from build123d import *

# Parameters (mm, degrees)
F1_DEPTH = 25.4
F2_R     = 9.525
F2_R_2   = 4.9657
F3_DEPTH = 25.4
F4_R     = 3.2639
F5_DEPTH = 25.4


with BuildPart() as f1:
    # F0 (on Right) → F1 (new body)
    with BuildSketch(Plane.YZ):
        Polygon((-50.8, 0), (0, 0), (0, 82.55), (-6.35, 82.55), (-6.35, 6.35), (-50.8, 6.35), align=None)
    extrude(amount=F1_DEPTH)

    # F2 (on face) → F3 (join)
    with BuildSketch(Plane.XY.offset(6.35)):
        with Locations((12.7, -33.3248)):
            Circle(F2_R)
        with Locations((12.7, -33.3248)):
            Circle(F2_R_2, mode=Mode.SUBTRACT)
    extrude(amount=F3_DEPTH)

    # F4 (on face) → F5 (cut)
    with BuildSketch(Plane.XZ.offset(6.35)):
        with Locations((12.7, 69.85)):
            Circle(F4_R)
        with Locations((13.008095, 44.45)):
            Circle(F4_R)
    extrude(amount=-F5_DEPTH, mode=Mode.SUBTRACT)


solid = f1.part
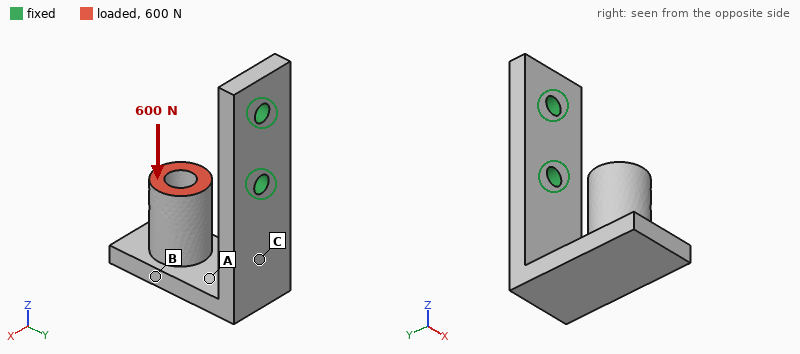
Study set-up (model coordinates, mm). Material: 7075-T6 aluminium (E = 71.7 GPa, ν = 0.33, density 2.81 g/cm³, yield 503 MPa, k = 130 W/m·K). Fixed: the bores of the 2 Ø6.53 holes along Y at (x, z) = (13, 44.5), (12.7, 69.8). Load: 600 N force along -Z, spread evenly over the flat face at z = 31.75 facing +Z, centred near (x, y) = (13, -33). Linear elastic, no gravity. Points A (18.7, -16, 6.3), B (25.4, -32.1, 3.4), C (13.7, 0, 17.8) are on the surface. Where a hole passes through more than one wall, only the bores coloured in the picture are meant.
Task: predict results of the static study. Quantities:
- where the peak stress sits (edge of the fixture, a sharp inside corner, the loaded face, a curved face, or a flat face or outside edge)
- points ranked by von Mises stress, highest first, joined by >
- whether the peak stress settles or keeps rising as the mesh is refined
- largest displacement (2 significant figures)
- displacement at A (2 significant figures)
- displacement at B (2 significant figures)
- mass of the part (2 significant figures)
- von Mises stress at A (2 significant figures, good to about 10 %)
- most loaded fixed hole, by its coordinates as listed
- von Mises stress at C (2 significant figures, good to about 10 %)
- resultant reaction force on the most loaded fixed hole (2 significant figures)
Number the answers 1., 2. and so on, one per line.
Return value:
1. edge of the fixture
2. C > A > B
3. keeps rising
4. 1.2 mm
5. 0.40 mm
6. 0.73 mm
7. 71 g
8. 59 MPa
9. (13, 44.5)
10. 94 MPa
11. 530 N
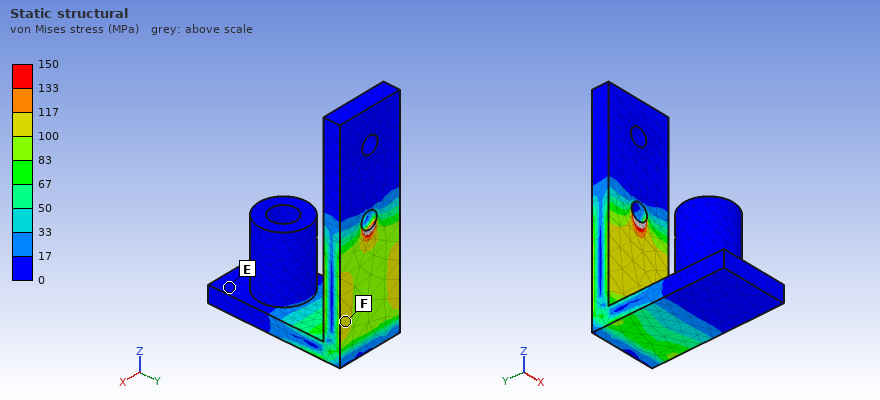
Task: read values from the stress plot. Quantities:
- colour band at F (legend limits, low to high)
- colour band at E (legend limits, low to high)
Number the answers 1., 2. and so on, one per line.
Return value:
1. 100 to 117 MPa
2. 0 to 17 MPa
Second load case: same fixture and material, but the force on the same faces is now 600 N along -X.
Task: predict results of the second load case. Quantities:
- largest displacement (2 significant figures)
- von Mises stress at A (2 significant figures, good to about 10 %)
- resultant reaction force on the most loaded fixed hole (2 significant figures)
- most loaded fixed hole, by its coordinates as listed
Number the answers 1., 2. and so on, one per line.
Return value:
1. 0.81 mm
2. 96 MPa
3. 760 N
4. (13, 44.5)
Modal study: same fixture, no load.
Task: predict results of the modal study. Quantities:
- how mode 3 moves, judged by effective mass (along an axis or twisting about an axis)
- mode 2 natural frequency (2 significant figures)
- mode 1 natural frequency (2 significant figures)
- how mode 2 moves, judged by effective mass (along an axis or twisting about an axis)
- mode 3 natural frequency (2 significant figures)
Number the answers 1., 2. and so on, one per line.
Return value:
1. along Y
2. 980 Hz
3. 720 Hz
4. along X
5. 1700 Hz
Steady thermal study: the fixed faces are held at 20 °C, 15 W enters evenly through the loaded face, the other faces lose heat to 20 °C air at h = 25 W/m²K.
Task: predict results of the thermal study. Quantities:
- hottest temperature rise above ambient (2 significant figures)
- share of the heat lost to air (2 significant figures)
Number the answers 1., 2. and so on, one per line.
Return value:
1. 46 K
2. 34 %
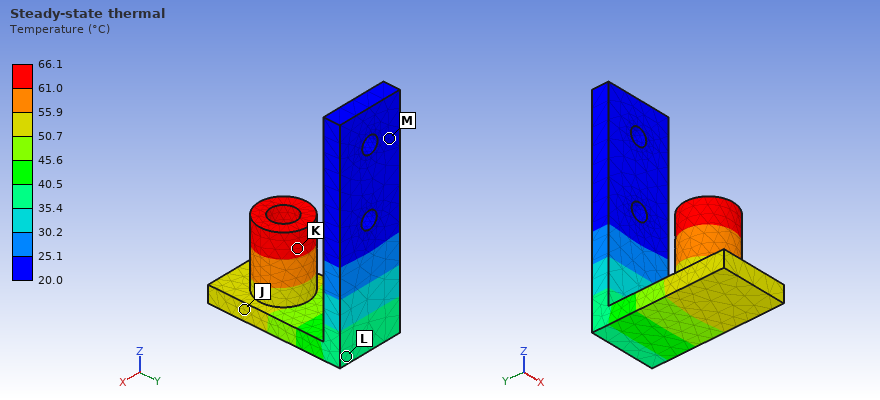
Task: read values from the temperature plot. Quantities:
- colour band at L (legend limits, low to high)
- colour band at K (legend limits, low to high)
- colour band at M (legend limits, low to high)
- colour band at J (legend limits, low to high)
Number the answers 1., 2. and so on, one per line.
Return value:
1. 35.4 to 40.5 °C
2. 61.0 to 66.1 °C
3. 20.0 to 25.1 °C
4. 50.7 to 55.9 °C
